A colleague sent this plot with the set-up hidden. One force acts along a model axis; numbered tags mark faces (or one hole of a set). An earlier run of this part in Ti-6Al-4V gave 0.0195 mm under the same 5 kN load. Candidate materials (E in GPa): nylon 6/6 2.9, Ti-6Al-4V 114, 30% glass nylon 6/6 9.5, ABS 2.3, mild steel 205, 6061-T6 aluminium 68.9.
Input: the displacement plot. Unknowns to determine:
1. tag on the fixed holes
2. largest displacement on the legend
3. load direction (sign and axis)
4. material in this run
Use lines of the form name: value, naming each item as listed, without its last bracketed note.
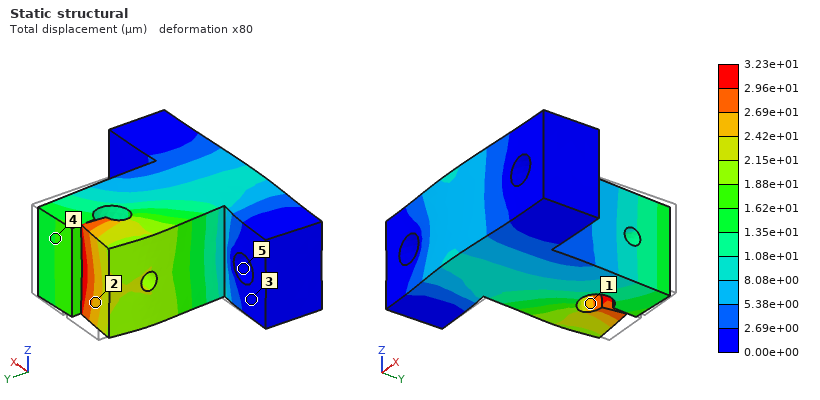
tag on the fixed holes: 5
largest displacement on the legend: 3.23e+01 µm
load direction: -Y
material in this run: 6061-T6 aluminium
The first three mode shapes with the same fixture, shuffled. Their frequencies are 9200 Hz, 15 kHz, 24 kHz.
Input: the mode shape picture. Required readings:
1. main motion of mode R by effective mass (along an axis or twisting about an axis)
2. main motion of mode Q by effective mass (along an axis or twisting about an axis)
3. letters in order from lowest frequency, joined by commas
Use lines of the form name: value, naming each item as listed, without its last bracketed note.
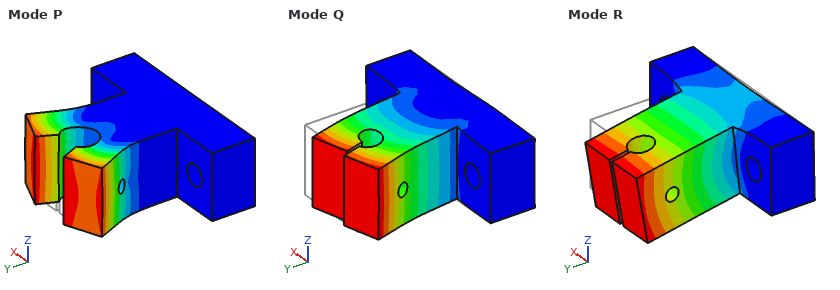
main motion of mode R by effective mass: along Z
main motion of mode Q by effective mass: along X
letters in order from lowest frequency, joined by commas: R, Q, P
